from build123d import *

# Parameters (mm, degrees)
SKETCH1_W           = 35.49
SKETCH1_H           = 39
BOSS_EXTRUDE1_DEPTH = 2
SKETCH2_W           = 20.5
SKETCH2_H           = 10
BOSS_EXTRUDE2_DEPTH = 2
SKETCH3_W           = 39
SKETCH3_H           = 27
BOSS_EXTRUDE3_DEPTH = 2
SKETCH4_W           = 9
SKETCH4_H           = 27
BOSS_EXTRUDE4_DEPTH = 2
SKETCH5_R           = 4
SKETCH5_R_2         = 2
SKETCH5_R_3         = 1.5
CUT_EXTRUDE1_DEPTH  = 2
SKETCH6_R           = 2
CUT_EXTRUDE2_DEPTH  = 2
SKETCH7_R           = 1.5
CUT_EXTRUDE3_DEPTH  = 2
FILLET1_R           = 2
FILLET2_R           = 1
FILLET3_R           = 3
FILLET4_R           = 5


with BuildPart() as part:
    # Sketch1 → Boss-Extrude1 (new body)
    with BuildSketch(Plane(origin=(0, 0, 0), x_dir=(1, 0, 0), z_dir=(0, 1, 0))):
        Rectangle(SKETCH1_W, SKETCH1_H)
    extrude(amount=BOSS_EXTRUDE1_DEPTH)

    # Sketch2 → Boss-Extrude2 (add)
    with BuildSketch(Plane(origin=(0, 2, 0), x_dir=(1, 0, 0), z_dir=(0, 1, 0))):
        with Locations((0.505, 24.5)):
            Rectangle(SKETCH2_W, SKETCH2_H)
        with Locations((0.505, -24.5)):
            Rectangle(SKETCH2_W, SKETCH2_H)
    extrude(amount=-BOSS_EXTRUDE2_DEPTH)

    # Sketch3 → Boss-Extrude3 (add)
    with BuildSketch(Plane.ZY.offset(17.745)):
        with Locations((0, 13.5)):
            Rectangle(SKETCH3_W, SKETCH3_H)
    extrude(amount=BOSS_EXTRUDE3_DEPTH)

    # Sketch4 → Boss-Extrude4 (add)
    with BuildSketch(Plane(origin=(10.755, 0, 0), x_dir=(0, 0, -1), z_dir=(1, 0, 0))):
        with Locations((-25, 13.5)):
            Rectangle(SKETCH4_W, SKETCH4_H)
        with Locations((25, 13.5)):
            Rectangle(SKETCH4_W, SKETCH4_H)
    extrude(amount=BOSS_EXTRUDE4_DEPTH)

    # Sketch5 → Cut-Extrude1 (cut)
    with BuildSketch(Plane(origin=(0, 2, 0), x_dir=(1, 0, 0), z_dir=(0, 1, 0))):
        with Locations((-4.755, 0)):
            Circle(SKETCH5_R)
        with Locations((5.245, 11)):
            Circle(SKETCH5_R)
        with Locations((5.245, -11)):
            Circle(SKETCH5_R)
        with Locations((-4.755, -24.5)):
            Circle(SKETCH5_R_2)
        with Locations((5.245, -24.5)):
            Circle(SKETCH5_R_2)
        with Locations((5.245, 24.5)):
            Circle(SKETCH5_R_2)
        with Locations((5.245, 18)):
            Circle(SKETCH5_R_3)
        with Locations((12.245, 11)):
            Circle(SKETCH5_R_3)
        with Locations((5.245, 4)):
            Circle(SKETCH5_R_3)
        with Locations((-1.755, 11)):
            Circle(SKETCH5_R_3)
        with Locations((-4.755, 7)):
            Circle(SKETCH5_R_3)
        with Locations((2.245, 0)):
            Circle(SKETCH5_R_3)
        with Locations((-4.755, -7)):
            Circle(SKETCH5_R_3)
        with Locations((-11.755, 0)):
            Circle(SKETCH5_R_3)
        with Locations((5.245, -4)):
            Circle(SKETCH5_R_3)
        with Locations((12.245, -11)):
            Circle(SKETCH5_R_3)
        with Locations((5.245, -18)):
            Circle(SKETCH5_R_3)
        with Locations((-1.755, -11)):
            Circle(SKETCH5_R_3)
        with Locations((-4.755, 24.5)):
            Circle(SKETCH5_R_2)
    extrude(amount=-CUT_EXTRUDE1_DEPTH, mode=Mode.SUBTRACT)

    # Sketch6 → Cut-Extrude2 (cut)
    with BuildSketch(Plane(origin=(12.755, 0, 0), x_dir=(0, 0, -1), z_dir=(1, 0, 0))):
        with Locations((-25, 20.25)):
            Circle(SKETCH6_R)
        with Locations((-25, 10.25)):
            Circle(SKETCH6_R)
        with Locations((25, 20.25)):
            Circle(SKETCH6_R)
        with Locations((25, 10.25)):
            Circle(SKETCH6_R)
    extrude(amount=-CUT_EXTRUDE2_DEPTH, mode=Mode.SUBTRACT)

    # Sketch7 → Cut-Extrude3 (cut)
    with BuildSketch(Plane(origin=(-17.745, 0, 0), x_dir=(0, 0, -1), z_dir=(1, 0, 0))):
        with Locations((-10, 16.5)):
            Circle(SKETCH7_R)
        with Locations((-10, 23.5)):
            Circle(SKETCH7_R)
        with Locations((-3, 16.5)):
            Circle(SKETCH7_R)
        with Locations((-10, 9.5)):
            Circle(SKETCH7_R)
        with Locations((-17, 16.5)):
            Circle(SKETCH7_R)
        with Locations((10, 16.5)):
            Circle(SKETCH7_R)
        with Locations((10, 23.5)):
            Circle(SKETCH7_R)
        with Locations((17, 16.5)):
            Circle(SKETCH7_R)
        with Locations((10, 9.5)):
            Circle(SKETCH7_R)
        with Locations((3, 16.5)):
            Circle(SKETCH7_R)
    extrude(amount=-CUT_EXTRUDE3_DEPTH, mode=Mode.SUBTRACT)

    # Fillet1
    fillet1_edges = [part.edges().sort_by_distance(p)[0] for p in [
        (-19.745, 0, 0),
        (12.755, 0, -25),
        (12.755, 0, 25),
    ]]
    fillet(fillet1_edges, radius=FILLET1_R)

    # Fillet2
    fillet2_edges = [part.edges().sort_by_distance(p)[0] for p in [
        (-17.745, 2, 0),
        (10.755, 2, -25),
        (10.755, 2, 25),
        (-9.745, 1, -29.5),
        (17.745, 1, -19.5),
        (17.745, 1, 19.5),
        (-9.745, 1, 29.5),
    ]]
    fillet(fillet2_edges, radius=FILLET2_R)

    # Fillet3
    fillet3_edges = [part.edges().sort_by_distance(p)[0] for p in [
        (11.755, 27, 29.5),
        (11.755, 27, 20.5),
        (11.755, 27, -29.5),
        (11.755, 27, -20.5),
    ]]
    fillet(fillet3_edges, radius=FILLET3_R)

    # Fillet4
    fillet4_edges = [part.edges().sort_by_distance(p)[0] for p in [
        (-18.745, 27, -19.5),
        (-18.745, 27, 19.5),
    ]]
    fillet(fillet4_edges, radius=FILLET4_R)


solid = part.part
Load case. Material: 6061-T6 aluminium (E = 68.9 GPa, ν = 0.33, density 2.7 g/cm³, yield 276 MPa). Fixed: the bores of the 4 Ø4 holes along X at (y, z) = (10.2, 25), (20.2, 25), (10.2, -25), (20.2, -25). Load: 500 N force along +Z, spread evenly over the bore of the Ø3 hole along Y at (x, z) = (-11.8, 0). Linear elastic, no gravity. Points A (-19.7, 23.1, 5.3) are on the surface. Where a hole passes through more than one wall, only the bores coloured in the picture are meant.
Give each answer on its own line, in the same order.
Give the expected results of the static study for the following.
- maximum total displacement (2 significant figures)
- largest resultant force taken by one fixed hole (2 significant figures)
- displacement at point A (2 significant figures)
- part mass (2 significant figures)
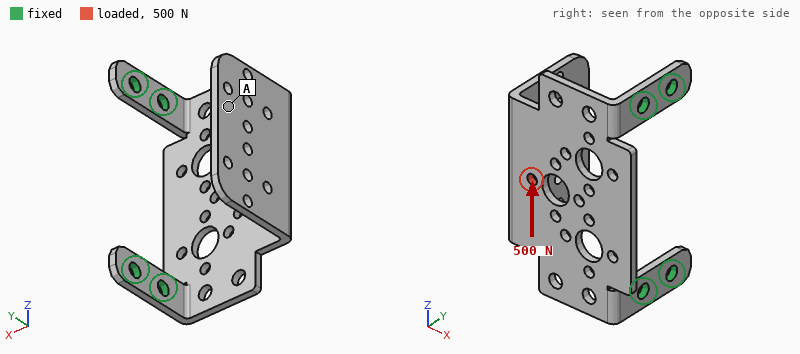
0.26 mm
380 N
0.23 mm
16 g
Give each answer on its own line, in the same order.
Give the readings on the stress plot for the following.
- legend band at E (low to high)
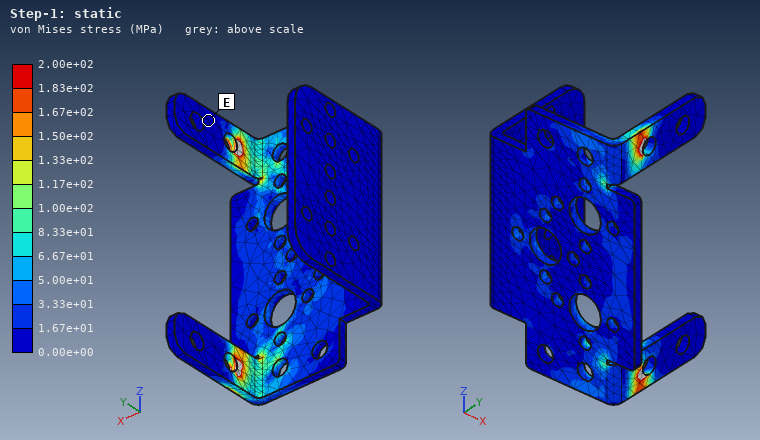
0.00e+00 to 1.67e+01 MPa
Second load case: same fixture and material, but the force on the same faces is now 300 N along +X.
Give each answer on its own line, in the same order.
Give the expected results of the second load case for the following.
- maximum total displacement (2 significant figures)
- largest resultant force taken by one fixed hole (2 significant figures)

0.40 mm
160 N
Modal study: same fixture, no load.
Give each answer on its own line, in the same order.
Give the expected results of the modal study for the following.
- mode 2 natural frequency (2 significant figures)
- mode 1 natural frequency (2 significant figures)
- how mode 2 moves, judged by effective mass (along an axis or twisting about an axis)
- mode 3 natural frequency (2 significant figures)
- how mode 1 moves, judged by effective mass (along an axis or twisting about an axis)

1200 Hz
430 Hz
along Z
1600 Hz
along Y
